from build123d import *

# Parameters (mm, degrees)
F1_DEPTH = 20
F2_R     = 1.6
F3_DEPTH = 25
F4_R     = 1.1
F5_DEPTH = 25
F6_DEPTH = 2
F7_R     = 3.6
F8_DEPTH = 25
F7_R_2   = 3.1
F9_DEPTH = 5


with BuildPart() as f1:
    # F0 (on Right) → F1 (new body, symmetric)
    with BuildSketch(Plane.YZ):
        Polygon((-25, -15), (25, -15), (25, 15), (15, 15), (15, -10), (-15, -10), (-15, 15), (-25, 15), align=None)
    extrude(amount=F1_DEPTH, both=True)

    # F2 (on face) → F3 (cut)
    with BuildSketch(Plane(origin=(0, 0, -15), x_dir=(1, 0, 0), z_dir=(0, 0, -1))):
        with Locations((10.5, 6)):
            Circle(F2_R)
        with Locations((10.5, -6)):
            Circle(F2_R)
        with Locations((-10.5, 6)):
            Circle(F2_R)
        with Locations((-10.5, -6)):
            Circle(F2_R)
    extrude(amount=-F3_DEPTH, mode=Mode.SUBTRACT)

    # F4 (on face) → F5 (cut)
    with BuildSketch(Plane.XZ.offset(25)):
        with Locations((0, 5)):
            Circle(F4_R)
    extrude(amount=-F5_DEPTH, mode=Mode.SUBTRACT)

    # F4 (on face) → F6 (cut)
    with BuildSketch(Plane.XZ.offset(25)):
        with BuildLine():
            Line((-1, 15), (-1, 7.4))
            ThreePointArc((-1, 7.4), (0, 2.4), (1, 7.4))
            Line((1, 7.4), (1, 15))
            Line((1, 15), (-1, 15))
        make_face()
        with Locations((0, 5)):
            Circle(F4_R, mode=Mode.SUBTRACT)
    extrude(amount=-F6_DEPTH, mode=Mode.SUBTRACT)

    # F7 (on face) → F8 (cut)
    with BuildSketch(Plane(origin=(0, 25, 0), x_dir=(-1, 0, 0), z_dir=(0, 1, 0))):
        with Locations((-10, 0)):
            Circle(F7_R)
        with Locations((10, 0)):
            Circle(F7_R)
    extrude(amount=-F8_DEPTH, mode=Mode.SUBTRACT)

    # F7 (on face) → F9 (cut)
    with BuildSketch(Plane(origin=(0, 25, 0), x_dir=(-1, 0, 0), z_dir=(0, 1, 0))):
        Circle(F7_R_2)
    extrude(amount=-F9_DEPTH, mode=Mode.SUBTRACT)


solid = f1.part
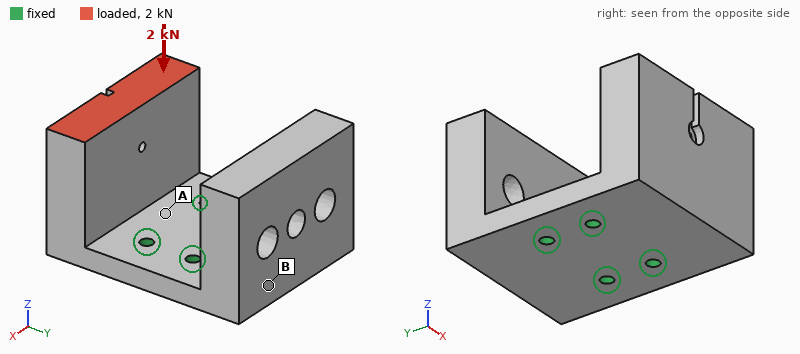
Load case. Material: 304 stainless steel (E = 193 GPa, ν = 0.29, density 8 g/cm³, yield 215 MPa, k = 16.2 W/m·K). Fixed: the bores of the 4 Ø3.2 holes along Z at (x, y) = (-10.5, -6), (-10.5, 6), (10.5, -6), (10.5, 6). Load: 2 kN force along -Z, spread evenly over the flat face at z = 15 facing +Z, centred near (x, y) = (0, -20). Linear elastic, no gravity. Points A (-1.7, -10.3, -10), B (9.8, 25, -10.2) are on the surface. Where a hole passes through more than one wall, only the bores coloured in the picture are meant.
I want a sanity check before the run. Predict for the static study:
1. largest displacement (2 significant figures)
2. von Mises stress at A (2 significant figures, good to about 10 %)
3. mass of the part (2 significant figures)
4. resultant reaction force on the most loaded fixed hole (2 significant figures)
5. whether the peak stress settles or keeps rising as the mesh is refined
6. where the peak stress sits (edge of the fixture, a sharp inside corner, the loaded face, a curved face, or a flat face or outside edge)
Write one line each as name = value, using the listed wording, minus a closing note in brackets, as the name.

largest displacement = 81 µm
von Mises stress at A = 86 MPa
mass of the part = 230 g
resultant reaction force on the most loaded fixed hole = 1.4 kN
whether the peak stress settles or keeps rising as the mesh is refined = keeps rising
where the peak stress sits = edge of the fixture
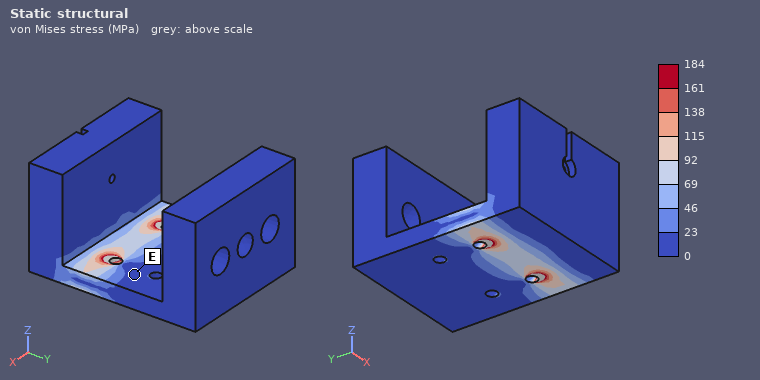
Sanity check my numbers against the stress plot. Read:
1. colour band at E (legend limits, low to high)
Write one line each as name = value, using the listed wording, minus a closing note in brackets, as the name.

colour band at E = 0 to 23 MPa
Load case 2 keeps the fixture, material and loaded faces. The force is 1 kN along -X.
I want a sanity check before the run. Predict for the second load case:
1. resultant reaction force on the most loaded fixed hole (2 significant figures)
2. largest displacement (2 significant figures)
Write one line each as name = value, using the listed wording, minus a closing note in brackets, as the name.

resultant reaction force on the most loaded fixed hole = 1.3 kN
largest displacement = 26 µm
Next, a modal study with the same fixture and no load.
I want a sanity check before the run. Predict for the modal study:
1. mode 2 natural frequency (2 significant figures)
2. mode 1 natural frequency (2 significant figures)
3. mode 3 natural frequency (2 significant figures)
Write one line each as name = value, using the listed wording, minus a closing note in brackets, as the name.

mode 2 natural frequency = 2400 Hz
mode 1 natural frequency = 2400 Hz
mode 3 natural frequency = 5200 Hz
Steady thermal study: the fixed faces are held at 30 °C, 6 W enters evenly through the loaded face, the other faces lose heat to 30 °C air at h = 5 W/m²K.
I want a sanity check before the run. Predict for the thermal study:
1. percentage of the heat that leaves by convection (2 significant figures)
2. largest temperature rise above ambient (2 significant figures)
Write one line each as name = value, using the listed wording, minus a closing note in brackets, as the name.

percentage of the heat that leaves by convection = 9.9 %
largest temperature rise above ambient = 46 K
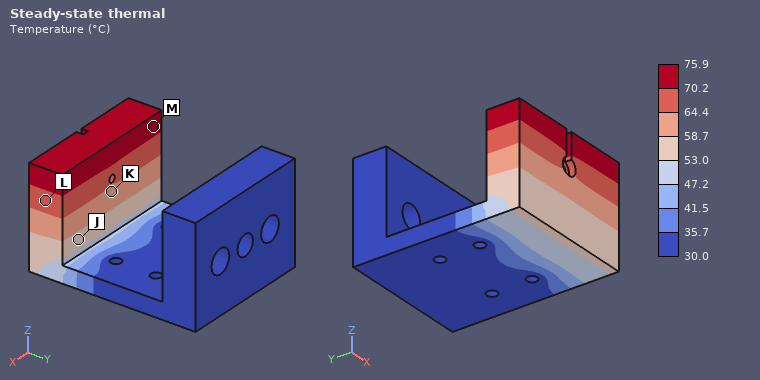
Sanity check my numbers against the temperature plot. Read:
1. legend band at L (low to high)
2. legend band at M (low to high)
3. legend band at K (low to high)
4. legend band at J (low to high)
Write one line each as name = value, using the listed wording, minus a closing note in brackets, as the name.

legend band at L = 64.4 to 70.2 °C
legend band at M = 70.2 to 75.9 °C
legend band at K = 58.7 to 64.4 °C
legend band at J = 53.0 to 58.7 °C
